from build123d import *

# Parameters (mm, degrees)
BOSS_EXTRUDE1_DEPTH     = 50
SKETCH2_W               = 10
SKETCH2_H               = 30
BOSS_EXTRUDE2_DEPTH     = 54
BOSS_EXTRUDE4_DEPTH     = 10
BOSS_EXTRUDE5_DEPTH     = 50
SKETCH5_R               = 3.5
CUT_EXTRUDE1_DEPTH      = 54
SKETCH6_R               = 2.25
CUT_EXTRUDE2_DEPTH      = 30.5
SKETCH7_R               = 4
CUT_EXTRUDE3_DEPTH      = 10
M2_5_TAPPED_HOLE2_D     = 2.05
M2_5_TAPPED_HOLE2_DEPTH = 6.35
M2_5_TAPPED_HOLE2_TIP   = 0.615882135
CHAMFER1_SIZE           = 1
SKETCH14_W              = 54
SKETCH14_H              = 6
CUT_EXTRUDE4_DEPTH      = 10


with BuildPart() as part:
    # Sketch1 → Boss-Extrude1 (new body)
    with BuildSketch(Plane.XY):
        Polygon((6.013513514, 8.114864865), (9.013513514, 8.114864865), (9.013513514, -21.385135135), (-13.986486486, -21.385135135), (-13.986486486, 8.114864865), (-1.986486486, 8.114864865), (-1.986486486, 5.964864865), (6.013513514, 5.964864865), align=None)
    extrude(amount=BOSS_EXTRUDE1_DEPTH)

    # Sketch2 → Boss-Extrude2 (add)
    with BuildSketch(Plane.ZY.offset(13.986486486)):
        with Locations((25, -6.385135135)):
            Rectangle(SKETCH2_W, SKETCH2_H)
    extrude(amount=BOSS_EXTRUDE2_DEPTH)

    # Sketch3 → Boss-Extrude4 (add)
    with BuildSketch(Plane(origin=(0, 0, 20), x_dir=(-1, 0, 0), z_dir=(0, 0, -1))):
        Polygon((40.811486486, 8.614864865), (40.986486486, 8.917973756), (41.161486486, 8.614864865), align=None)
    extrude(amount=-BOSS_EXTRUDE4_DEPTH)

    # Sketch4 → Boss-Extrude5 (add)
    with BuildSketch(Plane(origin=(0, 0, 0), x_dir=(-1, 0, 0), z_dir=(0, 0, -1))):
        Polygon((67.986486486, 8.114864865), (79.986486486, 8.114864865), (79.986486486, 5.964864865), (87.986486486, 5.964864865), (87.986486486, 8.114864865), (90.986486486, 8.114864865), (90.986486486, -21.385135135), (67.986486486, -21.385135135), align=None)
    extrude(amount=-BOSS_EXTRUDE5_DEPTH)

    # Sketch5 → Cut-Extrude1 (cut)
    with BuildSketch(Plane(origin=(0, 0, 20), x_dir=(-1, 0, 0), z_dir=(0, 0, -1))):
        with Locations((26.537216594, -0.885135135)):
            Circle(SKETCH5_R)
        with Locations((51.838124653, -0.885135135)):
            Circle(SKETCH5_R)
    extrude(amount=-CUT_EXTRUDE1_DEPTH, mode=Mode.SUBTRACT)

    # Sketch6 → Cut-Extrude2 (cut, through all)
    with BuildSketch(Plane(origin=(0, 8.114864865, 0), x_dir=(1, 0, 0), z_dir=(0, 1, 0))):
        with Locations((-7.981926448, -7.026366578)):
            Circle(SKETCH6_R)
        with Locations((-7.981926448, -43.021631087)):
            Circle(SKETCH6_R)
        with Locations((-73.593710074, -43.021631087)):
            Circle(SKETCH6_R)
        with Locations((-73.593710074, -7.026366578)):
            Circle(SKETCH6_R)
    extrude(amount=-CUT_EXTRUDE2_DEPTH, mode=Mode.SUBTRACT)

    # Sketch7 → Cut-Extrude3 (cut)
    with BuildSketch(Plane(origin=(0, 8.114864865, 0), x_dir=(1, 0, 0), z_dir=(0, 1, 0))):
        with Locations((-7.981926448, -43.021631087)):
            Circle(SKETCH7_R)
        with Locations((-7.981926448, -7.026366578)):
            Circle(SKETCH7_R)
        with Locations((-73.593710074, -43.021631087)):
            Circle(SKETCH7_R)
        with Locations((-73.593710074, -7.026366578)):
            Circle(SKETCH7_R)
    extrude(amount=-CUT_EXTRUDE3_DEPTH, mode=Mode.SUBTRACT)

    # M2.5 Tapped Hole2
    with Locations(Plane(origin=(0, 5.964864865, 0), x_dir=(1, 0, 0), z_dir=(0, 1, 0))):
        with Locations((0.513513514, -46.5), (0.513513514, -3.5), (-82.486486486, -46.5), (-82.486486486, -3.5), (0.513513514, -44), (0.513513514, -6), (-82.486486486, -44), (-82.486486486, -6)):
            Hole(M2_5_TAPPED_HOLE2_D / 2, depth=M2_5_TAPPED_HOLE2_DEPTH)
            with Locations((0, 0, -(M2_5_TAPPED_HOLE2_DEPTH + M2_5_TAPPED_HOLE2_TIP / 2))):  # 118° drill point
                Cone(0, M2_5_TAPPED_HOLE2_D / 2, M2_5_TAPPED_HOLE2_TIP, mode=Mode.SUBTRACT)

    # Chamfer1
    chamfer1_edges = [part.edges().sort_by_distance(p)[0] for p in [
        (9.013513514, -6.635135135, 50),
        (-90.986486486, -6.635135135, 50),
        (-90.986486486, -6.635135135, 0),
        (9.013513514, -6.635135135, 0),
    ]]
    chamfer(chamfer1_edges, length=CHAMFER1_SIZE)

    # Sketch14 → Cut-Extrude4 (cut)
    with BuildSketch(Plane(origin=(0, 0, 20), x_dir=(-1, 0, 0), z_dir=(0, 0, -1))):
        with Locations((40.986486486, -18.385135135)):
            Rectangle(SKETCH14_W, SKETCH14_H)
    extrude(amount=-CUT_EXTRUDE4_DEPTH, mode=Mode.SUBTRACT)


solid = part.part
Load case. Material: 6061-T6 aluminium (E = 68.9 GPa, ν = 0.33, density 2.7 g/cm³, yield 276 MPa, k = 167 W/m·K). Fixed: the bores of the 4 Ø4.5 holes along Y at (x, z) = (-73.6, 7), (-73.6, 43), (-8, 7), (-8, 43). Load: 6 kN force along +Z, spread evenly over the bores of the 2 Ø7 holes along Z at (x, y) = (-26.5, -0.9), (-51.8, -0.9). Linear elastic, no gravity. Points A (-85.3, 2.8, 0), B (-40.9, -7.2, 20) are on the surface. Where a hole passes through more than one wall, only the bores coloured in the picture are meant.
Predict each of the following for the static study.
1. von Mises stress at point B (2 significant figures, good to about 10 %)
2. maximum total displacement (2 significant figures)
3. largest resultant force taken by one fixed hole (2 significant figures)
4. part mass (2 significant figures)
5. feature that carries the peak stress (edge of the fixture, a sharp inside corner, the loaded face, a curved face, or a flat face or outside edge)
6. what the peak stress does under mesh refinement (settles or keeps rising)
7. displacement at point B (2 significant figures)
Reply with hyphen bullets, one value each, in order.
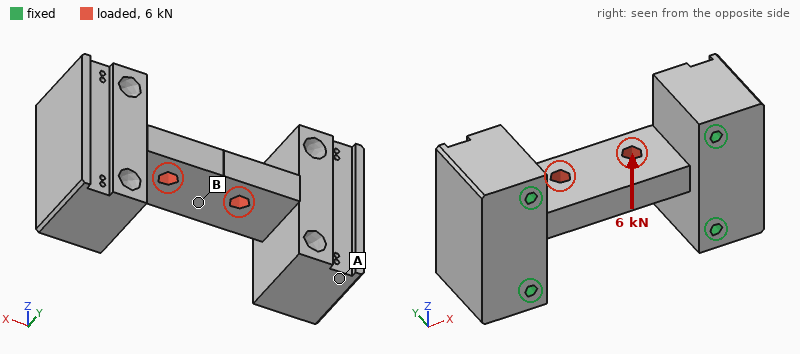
- 32 MPa
- 53 µm
- 2.2 kN
- 200 g
- a sharp inside corner
- keeps rising
- 38 µm
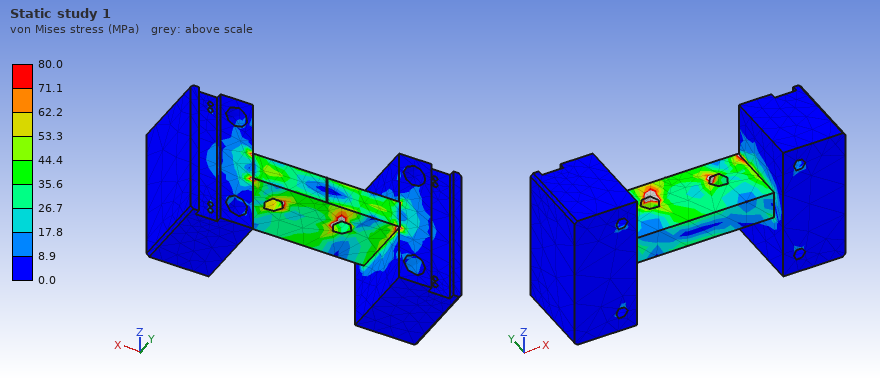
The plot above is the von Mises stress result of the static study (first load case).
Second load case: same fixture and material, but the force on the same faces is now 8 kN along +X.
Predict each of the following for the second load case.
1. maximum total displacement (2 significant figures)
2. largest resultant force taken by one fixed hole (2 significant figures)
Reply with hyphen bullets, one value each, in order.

- 11 µm
- 2.1 kN
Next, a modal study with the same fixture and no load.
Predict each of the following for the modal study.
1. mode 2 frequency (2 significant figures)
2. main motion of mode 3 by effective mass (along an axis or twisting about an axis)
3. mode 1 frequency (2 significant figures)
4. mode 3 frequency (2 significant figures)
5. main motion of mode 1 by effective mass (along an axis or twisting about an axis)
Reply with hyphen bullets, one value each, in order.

- 14 kHz
- along X
- 12 kHz
- 17 kHz
- along Z
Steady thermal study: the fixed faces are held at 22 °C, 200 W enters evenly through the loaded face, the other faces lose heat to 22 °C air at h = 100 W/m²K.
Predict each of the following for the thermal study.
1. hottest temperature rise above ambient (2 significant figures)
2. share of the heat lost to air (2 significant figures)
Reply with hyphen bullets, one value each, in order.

- 63 K
- 11 %
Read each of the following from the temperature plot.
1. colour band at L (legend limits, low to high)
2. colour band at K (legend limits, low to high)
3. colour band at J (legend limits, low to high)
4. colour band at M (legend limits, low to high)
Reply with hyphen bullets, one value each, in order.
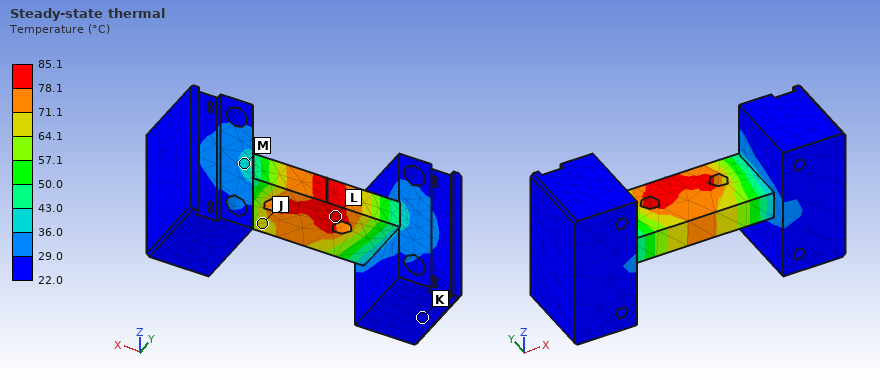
- 78.1 to 85.1 °C
- 22.0 to 29.0 °C
- 64.1 to 71.1 °C
- 36.0 to 43.0 °C
